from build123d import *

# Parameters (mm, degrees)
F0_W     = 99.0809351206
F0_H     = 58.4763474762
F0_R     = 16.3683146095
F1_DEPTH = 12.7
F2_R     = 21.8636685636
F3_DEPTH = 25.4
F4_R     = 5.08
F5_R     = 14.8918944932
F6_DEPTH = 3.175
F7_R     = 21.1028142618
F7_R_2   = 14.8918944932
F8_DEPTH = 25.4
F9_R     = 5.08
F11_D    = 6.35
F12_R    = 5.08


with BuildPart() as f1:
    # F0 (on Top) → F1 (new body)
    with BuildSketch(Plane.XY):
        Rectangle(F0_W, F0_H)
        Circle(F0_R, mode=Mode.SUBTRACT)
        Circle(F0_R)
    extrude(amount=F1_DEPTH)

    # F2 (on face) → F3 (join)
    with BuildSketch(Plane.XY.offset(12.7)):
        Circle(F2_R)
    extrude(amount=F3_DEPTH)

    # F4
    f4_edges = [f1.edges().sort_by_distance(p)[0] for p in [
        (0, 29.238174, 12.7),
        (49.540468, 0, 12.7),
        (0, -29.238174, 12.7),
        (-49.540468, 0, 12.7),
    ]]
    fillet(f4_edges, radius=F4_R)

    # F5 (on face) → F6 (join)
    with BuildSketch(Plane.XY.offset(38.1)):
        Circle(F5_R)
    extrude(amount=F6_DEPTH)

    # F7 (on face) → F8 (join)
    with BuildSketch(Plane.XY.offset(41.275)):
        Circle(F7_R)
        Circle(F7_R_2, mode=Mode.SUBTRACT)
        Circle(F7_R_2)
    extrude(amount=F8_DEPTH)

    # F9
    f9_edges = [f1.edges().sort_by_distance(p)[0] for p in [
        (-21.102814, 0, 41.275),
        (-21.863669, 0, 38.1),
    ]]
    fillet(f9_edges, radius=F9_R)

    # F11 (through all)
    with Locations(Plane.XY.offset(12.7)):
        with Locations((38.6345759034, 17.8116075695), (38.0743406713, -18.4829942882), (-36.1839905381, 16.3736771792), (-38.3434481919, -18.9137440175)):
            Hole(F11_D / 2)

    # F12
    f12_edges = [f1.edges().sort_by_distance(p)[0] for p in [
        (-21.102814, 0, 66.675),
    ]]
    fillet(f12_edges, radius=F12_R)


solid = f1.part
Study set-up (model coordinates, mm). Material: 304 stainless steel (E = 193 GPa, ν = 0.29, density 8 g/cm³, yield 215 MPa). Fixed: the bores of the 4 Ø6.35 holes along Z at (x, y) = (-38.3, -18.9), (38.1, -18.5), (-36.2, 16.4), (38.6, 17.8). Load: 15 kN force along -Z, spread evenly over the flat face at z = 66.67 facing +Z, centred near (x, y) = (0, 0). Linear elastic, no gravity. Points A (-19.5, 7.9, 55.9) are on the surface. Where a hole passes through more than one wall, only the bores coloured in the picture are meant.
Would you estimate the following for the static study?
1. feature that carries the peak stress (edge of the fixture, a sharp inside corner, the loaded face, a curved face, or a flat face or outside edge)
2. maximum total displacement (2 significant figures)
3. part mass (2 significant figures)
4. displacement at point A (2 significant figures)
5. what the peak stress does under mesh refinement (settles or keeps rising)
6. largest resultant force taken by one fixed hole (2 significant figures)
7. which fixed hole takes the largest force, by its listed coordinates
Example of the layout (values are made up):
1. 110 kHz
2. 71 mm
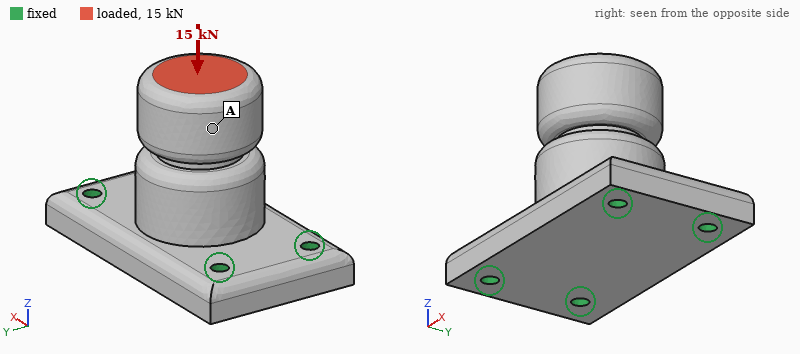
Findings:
1. edge of the fixture
2. 16 µm
3. 1.2 kg
4. 14 µm
5. keeps rising
6. 4.5 kN
7. (-36.2, 16.4)
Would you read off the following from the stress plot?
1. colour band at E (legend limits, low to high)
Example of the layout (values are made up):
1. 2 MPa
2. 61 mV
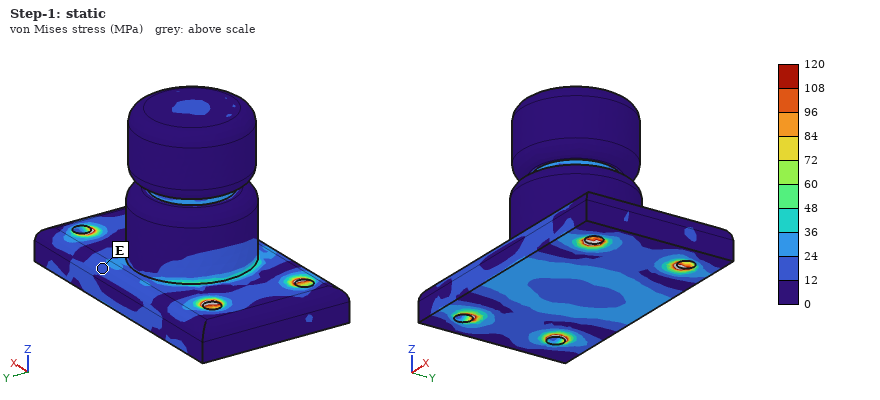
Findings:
1. 12 to 24 MPa
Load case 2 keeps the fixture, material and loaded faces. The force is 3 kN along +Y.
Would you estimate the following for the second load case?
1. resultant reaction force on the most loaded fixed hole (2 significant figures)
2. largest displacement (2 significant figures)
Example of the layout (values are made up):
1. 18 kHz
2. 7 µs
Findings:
1. 2.6 kN
2. 36 µm
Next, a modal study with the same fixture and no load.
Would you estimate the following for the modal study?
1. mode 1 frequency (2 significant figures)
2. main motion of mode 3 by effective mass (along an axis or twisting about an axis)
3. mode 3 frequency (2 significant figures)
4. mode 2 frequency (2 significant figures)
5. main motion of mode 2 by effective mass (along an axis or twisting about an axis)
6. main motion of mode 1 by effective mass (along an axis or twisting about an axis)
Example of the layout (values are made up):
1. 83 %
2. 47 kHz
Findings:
1. 3200 Hz
2. along Z
3. 6100 Hz
4. 4600 Hz
5. along X
6. along Y
